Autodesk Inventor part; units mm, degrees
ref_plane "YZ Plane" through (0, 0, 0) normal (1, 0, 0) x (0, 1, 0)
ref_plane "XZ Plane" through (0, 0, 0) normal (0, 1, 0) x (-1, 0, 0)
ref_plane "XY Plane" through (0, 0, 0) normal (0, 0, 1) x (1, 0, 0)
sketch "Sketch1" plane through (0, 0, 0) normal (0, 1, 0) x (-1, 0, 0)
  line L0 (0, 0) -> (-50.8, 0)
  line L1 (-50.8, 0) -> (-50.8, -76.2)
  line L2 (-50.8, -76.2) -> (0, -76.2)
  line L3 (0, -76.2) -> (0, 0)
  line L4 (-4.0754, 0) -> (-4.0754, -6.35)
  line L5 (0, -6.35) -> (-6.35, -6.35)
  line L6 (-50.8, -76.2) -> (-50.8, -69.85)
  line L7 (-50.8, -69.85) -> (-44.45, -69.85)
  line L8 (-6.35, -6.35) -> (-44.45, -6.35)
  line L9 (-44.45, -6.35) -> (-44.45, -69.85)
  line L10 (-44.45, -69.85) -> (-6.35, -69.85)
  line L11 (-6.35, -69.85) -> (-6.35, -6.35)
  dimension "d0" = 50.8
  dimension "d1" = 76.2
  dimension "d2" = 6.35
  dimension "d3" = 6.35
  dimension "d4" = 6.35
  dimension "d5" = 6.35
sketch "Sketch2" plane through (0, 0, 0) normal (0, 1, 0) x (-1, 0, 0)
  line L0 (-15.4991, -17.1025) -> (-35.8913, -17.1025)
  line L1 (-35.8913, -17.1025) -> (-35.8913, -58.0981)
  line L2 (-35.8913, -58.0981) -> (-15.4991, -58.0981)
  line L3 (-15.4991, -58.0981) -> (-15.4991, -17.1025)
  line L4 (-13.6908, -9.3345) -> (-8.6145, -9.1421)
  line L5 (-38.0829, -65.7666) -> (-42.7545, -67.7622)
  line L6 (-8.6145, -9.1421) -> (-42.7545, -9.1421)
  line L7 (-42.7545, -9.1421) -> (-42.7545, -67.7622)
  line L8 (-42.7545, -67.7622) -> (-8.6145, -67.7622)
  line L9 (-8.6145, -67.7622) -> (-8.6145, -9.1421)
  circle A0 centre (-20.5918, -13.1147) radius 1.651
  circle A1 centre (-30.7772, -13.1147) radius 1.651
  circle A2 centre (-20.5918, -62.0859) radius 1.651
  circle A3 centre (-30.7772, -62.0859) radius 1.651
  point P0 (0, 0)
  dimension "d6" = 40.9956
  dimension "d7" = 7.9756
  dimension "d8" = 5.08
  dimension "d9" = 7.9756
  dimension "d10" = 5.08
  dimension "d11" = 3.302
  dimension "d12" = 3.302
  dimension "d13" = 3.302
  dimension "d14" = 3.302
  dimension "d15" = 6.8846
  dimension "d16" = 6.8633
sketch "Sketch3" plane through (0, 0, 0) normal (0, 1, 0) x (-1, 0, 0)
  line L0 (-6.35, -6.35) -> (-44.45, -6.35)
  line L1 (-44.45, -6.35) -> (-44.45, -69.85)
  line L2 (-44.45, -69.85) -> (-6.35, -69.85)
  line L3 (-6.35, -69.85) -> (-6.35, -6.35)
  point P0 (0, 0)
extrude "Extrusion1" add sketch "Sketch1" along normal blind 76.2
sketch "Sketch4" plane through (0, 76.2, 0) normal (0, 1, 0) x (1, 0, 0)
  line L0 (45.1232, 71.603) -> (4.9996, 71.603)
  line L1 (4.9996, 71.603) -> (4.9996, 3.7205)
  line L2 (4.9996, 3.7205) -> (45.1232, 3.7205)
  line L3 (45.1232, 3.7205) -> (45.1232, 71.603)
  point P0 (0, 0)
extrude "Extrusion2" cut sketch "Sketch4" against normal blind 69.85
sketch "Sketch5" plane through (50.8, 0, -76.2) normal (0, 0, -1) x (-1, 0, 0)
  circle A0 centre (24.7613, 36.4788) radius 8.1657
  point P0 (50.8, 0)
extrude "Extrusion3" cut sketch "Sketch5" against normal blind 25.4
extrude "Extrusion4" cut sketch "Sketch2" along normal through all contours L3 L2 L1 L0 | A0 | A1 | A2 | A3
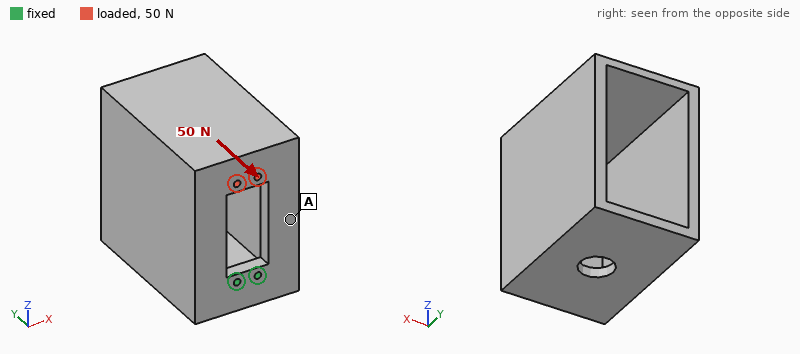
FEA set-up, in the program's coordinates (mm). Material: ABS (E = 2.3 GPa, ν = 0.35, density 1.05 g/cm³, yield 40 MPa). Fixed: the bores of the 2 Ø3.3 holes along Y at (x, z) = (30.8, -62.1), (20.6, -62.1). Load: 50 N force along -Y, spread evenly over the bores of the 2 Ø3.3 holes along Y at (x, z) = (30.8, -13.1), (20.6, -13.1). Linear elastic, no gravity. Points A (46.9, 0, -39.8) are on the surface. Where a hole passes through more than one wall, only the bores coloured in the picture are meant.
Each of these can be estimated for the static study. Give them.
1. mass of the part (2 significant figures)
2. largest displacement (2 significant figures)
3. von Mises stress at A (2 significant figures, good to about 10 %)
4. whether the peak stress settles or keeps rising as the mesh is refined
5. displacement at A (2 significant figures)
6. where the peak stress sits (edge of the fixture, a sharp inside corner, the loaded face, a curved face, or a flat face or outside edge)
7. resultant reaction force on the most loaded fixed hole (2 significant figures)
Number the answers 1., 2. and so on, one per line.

1. 100 g
2. 1.4 mm
3. 1.0 MPa
4. keeps rising
5. 0.37 mm
6. edge of the fixture
7. 30 N
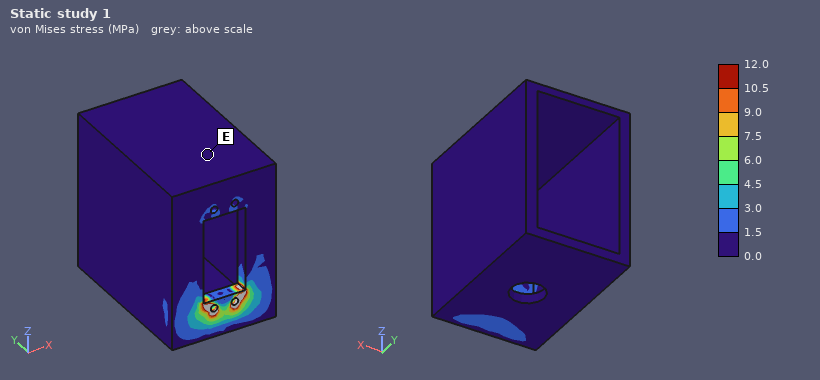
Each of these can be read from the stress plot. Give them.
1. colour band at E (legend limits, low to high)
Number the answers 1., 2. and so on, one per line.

1. 0.0 to 1.5 MPa
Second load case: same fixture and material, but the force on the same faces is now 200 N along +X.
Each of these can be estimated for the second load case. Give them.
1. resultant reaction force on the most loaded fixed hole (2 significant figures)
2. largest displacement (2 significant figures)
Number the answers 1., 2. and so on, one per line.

1. 690 N
2. 1.2 mm
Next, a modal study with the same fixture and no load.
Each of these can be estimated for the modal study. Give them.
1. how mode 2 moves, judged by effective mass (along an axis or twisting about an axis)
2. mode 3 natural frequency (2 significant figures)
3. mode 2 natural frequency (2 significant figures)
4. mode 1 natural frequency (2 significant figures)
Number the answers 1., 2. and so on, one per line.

1. along X
2. 400 Hz
3. 220 Hz
4. 120 Hz
